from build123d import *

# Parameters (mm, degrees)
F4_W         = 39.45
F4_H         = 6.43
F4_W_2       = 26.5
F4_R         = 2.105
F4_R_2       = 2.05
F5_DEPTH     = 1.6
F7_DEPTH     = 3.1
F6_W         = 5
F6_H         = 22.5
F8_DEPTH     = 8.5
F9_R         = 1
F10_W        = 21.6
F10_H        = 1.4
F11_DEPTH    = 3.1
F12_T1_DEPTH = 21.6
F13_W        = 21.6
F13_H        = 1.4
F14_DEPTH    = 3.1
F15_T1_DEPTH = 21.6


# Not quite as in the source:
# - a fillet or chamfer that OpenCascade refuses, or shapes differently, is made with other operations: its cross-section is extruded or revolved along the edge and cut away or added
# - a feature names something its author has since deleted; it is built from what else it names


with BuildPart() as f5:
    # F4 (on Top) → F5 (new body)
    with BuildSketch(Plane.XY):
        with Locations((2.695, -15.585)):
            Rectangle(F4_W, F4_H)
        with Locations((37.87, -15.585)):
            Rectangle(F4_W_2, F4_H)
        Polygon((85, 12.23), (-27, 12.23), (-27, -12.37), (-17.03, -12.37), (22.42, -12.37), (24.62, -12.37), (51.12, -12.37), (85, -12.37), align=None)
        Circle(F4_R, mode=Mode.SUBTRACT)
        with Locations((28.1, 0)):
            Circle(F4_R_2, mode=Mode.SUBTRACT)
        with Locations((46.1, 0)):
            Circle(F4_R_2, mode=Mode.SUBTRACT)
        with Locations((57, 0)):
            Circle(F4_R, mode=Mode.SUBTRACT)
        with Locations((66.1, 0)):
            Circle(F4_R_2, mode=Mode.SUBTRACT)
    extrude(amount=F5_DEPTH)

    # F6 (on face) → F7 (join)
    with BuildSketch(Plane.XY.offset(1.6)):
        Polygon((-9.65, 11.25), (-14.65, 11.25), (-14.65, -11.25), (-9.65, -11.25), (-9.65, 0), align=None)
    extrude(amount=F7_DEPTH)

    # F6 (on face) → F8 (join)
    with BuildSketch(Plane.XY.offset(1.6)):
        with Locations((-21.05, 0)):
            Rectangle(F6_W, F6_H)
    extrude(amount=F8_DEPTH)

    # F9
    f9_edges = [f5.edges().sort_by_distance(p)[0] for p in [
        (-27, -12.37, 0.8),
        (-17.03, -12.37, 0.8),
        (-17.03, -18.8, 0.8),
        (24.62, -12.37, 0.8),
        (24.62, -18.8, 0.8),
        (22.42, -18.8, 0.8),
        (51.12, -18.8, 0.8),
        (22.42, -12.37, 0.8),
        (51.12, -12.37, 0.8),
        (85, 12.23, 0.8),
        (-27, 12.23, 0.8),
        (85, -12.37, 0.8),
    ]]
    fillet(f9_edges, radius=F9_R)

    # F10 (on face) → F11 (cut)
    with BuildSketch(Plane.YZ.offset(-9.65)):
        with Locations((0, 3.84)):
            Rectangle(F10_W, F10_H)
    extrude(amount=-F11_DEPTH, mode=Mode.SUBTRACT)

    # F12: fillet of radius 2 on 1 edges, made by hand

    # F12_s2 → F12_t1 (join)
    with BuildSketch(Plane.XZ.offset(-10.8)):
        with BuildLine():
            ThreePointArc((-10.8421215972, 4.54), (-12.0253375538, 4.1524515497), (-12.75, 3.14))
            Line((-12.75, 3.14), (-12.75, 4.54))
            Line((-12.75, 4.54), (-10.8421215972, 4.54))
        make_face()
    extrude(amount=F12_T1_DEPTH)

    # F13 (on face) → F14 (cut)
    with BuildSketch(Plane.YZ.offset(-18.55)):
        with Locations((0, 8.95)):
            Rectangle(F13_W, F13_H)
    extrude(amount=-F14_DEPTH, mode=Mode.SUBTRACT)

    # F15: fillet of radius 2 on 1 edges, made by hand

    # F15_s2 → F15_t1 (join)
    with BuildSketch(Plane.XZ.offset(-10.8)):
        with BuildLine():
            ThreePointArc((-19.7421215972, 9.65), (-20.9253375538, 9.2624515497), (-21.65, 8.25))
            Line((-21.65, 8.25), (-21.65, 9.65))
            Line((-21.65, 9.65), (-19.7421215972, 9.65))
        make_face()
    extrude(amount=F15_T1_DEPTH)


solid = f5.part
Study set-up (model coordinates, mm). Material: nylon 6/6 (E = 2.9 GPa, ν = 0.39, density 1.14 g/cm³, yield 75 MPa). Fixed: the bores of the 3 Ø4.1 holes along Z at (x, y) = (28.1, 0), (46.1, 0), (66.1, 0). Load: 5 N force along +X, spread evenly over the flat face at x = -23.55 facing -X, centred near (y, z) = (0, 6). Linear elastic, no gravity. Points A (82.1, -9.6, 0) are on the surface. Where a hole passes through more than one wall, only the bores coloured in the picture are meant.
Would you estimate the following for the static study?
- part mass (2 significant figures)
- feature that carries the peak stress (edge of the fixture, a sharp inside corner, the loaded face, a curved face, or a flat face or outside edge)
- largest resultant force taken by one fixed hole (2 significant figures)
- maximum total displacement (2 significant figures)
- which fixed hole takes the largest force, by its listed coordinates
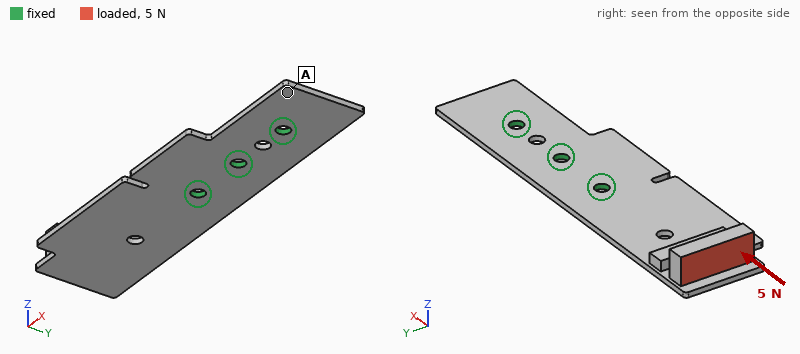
7.0 g
a flat face or outside edge
3.8 N
1.2 mm
(28.1, 0)
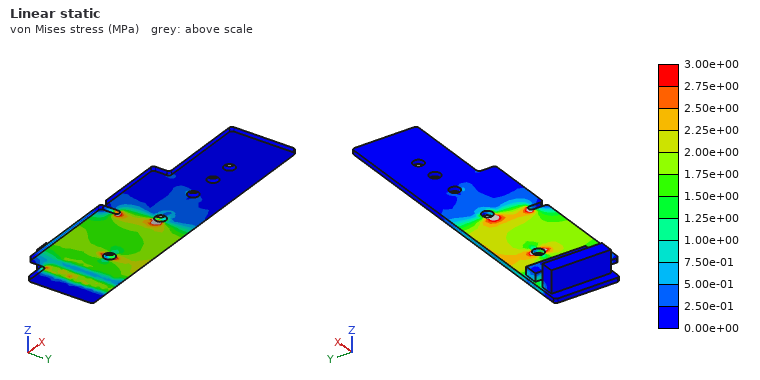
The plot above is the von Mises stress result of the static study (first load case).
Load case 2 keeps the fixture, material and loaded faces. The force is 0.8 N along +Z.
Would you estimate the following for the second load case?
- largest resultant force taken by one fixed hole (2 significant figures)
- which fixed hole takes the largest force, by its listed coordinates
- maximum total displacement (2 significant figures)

1.4 N
(28.1, 0)
1.3 mm
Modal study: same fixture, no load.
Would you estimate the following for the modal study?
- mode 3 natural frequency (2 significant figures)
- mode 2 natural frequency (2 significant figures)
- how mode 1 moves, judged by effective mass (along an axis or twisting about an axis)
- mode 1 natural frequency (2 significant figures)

720 Hz
370 Hz
along Z
95 Hz
